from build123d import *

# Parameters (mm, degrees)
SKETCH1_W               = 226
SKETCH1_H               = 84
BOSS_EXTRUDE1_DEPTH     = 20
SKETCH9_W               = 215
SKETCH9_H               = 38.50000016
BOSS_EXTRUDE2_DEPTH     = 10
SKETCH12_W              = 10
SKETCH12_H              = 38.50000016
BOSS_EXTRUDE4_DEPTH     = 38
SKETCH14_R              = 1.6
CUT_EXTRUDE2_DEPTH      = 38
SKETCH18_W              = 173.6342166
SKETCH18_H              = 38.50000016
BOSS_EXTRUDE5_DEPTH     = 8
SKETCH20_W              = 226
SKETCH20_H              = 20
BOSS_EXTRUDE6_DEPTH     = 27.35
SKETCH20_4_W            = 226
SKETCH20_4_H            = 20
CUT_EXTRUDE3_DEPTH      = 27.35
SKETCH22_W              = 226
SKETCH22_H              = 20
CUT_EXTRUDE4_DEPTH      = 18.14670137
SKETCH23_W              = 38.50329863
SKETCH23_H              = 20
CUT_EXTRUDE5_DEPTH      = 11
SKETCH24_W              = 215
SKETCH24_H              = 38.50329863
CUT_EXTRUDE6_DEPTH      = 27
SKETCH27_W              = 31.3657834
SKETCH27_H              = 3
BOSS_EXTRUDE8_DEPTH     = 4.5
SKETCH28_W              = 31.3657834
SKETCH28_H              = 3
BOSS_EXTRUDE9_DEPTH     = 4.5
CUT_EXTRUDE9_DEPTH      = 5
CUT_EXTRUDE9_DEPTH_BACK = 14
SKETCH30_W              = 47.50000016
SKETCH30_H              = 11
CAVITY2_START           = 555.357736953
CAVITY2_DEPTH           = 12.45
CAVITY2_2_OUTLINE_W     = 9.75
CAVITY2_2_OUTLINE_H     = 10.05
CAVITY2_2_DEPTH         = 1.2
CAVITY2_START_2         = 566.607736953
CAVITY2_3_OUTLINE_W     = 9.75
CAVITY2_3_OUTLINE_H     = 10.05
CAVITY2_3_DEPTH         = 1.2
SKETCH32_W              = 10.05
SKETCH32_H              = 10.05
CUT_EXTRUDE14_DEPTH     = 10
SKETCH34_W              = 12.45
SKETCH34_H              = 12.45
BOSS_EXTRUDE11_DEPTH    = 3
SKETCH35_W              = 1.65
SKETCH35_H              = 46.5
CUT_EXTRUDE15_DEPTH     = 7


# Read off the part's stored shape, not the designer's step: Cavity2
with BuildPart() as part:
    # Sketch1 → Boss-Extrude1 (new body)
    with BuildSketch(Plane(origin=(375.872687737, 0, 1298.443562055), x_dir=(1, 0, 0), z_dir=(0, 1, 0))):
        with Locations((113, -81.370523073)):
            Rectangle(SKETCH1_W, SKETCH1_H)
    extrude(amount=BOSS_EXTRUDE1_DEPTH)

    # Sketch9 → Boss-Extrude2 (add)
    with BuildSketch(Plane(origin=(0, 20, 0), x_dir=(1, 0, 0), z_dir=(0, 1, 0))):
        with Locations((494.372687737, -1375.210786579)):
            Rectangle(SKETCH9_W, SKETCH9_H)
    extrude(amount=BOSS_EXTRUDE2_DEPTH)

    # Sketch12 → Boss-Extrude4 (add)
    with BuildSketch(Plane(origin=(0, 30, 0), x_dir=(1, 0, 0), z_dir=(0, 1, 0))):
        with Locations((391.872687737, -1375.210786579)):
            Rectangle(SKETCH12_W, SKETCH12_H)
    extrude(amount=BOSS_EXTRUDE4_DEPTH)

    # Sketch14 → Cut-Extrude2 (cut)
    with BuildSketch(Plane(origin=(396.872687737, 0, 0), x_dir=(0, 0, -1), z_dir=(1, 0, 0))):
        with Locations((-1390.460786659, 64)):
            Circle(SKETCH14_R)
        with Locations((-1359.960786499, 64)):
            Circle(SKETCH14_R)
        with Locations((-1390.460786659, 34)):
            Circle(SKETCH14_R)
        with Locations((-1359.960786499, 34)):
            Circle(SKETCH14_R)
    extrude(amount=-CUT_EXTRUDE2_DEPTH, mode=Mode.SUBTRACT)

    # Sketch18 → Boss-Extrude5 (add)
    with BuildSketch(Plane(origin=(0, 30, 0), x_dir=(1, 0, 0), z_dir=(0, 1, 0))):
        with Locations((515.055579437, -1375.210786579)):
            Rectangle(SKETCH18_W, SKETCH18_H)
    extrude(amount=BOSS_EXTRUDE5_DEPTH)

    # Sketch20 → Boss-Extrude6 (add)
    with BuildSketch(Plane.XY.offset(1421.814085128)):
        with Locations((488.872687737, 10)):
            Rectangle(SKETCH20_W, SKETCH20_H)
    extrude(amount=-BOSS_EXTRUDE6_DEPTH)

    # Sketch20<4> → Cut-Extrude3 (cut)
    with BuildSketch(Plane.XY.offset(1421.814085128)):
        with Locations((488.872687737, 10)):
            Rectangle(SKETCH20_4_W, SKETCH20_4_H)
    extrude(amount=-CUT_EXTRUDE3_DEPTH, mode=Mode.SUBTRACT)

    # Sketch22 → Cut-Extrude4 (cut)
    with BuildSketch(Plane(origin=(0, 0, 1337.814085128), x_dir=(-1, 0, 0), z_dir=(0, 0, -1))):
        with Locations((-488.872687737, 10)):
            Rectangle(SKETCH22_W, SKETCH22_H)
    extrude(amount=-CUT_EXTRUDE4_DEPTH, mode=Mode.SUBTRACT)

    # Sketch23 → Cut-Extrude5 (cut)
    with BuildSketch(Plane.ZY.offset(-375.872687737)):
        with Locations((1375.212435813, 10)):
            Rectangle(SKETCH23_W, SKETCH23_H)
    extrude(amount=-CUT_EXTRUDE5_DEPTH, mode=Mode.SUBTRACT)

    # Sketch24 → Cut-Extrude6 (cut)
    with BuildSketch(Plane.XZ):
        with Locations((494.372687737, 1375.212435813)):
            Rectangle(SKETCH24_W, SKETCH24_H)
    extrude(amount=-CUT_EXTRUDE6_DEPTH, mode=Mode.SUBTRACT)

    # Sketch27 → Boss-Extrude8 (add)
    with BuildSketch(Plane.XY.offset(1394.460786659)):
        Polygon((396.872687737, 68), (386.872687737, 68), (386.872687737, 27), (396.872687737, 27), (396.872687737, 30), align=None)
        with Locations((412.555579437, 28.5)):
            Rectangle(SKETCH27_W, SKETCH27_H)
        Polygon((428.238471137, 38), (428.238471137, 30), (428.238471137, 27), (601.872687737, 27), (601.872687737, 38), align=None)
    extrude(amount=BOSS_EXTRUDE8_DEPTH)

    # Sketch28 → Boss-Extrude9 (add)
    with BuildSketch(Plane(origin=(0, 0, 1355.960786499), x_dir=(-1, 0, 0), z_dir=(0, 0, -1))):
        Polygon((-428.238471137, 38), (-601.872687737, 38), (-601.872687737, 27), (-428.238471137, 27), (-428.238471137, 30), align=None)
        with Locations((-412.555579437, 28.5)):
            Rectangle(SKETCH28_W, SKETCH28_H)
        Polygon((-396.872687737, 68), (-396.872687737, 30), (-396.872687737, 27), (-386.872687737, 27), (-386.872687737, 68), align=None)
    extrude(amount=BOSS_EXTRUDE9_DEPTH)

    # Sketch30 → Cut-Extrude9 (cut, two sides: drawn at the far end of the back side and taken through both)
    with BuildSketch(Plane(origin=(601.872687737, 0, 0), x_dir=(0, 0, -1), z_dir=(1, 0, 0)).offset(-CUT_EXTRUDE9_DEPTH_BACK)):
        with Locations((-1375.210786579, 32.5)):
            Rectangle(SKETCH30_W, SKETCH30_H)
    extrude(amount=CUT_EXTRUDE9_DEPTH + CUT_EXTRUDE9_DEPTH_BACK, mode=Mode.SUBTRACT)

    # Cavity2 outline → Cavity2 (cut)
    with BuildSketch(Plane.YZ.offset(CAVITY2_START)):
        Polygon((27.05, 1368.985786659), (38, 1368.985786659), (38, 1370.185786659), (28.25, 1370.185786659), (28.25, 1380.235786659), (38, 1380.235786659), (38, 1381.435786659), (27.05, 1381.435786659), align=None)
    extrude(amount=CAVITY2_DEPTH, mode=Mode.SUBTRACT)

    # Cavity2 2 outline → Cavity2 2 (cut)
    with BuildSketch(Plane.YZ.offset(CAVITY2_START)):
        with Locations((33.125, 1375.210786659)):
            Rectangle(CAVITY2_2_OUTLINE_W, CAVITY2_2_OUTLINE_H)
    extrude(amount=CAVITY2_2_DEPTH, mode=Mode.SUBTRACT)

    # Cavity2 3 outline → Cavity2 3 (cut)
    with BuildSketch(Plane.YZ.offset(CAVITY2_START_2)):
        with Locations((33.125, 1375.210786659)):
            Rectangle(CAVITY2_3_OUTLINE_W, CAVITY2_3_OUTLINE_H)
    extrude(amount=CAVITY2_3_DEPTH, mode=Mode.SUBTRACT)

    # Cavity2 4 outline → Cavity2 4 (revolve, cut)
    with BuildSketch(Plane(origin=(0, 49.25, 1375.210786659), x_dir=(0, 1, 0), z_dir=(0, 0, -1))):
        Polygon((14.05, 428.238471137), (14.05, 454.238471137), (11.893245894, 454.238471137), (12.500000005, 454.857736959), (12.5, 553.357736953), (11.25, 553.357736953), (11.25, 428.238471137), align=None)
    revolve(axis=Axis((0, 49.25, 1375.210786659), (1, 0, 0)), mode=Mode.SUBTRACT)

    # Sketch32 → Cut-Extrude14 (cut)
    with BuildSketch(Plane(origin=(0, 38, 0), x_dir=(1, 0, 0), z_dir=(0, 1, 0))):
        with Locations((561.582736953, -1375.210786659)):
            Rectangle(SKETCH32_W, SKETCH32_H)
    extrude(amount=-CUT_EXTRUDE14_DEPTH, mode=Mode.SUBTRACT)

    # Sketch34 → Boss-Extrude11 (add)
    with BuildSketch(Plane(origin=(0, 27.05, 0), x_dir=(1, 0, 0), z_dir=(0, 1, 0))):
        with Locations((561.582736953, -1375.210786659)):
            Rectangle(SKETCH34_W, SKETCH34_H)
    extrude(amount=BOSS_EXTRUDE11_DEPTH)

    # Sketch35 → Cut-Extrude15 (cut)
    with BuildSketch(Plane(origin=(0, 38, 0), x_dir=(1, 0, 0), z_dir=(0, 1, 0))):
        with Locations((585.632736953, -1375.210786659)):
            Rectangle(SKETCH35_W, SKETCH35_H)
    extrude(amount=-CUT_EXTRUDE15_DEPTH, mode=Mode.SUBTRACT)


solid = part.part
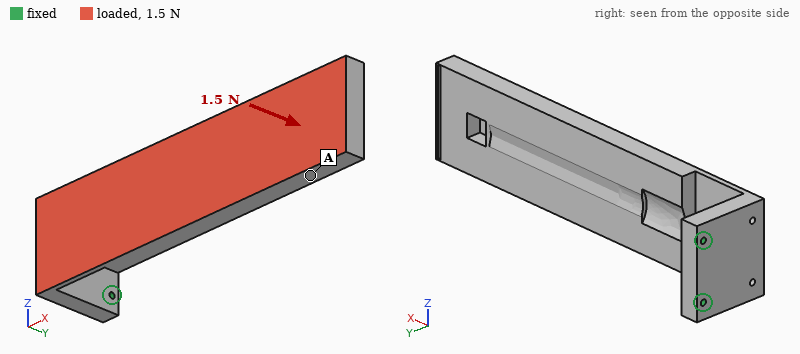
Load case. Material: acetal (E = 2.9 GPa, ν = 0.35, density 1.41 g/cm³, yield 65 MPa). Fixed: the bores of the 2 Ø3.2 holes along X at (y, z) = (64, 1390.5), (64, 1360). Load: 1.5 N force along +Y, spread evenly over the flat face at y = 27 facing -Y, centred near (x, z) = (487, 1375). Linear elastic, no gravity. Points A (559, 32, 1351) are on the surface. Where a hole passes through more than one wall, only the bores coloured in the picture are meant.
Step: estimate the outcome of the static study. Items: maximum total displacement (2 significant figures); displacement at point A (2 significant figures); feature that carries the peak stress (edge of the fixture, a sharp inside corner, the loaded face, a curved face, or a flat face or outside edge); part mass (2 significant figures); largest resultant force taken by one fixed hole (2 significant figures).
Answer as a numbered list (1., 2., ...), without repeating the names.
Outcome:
1. 2.2 mm
2. 1.8 mm
3. the loaded face
4. 150 g
5. 0.86 N
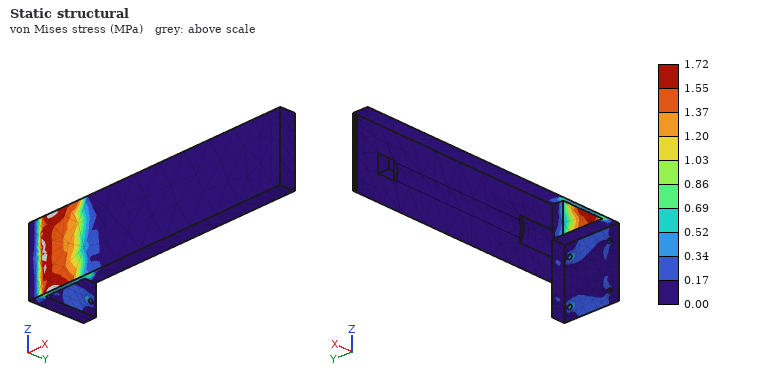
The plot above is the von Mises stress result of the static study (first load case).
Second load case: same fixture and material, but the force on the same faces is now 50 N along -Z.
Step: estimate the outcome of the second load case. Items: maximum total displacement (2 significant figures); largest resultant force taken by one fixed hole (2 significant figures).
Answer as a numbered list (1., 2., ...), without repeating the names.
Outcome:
1. 2.3 mm
2. 150 N
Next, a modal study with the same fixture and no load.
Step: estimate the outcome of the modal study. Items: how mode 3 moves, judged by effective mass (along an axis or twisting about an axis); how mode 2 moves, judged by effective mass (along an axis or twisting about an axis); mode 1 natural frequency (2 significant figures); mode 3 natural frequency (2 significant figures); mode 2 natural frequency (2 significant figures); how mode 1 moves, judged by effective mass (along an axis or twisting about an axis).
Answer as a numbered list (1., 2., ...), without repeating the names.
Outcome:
1. twisting about X
2. along Z
3. 14 Hz
4. 180 Hz
5. 76 Hz
6. along Y
